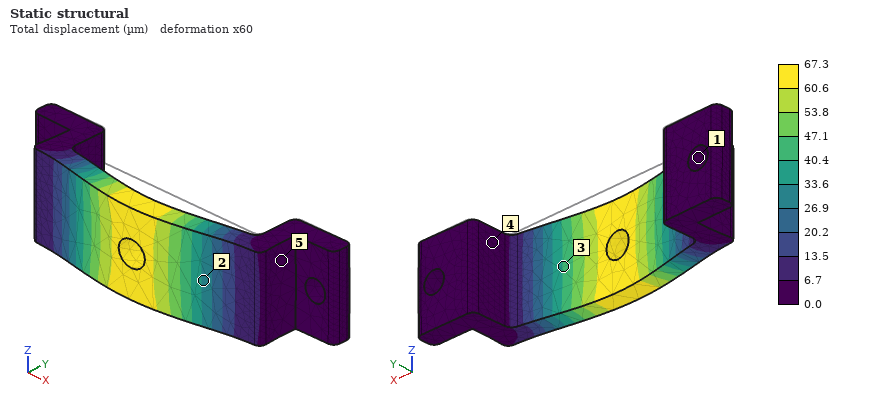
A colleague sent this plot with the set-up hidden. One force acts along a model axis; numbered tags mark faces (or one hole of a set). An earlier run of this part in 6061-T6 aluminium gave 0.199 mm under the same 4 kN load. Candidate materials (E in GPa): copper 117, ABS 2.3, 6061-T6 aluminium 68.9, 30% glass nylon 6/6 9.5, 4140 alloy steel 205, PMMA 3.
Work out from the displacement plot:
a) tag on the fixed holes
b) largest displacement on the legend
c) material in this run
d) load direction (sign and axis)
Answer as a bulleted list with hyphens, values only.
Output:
- 1
- 67.3 µm
- 4140 alloy steel
- -Y
